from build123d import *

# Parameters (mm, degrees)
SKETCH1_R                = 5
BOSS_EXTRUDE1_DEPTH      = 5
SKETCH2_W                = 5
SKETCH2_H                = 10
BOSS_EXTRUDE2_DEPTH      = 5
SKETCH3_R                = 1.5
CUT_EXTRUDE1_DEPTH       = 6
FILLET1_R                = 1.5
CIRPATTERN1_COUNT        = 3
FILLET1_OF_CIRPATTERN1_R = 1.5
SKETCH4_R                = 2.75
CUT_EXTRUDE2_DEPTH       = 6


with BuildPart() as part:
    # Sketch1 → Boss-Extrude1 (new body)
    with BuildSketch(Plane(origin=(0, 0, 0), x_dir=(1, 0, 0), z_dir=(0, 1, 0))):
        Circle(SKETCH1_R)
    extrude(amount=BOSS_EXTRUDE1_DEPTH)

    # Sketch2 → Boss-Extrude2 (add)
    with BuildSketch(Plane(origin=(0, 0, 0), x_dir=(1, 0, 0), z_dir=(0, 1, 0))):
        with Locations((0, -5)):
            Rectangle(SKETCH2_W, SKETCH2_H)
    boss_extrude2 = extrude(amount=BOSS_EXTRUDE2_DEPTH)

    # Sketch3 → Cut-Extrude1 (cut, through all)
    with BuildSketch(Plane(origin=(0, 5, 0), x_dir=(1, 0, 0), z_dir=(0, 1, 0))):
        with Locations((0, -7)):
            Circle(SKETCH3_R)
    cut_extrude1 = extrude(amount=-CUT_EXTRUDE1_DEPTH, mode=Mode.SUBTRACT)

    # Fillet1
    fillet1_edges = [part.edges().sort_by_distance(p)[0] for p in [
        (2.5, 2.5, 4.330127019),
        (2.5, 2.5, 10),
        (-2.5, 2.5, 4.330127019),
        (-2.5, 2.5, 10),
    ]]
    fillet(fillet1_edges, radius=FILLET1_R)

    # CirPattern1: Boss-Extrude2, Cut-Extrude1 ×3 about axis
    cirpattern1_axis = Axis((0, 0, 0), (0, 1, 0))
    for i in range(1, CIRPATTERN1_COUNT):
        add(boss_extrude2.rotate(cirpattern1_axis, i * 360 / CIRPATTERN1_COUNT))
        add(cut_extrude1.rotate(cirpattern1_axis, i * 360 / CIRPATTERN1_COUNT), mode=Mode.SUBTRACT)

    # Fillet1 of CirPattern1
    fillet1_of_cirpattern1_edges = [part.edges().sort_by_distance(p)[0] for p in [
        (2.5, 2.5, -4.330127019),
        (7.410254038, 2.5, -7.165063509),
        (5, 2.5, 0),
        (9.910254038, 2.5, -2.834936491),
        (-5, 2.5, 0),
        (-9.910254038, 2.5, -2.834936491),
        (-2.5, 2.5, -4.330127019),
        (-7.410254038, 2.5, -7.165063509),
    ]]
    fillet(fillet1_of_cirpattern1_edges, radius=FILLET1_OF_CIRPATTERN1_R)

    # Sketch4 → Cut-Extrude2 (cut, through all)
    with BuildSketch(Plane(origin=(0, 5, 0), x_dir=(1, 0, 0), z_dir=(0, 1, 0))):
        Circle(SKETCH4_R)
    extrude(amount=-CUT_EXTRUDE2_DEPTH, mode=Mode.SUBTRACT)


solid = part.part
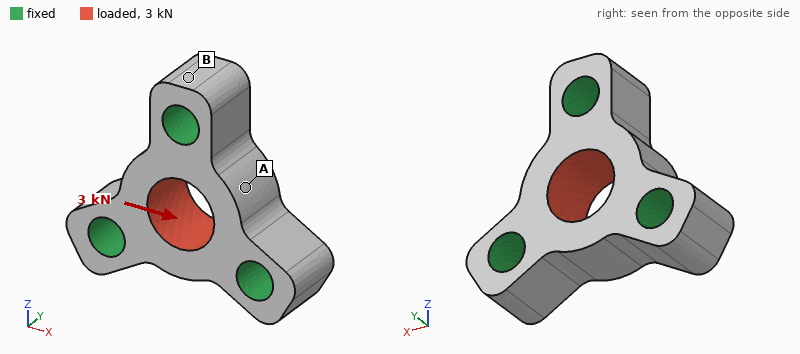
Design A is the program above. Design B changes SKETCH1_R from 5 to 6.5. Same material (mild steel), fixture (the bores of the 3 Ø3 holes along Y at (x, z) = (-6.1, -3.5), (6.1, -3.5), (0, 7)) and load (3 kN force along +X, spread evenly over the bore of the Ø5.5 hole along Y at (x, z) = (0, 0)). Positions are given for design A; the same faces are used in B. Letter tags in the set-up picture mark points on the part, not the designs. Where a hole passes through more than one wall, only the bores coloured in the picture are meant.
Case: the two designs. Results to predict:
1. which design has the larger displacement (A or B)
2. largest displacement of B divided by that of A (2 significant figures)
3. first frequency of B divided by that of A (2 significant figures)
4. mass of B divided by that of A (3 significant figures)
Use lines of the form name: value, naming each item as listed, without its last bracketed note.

which design has the larger displacement: A
largest displacement of B divided by that of A: 0.67
first frequency of B divided by that of A: 0.94
mass of B divided by that of A: 1.28
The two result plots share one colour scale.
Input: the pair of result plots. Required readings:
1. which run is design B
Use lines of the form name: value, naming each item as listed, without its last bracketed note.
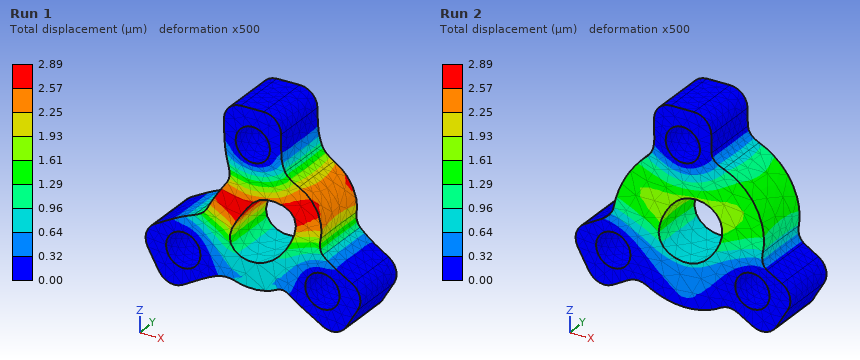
which run is design B: Run 2
